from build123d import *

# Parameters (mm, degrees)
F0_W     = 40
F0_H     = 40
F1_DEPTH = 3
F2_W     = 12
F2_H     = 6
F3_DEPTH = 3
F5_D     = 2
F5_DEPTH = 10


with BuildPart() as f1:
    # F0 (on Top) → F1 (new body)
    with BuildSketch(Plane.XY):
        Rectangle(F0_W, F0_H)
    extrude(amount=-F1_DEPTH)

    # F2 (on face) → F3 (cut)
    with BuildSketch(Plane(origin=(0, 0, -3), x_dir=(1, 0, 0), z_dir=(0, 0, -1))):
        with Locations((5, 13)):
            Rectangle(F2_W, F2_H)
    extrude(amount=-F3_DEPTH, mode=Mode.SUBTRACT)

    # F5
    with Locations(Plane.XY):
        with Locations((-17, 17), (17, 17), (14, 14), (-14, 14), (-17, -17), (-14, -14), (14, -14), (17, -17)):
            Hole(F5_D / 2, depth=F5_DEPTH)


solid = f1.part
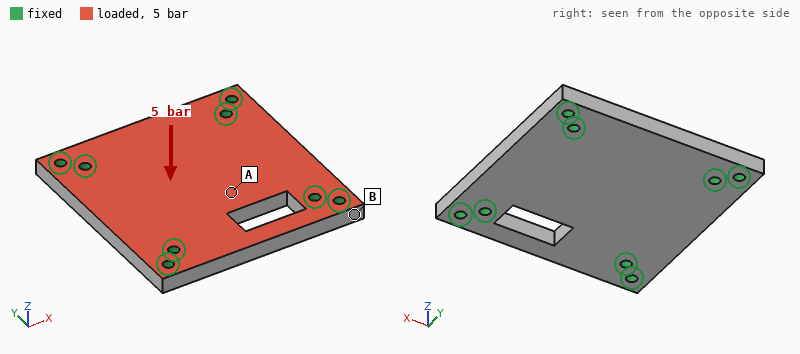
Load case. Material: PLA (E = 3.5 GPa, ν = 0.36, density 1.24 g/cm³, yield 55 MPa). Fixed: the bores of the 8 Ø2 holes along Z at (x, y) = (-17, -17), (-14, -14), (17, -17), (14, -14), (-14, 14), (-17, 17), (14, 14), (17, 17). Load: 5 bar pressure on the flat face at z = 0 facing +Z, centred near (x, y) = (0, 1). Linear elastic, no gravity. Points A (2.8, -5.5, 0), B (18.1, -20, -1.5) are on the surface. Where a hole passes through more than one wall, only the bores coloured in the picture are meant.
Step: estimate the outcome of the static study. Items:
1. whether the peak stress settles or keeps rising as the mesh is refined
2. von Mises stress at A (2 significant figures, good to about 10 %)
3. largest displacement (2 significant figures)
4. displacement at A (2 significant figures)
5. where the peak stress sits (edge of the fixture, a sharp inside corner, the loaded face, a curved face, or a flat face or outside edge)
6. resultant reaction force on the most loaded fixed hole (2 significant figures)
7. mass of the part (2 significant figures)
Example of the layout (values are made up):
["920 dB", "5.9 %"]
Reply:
["keeps rising", "12 MPa", "0.27 mm", "0.26 mm", "edge of the fixture", "210 N", "5.6 g"]
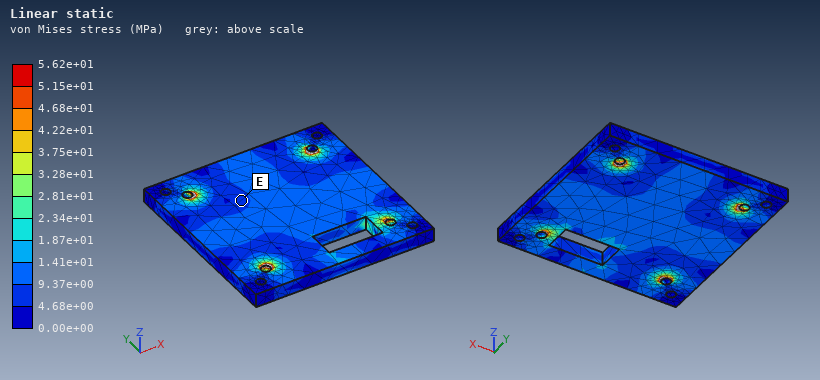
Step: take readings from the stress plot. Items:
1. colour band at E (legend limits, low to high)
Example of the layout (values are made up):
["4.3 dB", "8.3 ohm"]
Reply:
["4.68e+00 to 9.37e+00 MPa"]
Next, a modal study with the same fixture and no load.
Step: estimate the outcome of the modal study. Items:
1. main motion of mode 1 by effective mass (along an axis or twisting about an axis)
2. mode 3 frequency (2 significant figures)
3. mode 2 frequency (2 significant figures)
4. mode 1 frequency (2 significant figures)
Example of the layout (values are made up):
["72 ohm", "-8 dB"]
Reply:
["along Z", "6300 Hz", "6200 Hz", "4300 Hz"]
